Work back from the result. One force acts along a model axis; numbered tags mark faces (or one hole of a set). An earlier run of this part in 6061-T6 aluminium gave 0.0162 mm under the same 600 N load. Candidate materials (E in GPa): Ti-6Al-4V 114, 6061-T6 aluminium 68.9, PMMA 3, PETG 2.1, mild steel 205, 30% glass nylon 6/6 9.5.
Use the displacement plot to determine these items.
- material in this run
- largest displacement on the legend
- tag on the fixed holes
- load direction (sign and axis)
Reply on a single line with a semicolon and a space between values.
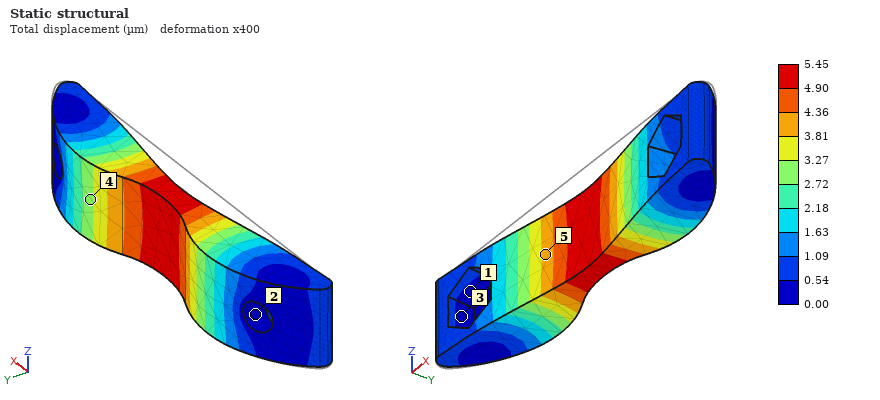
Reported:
mild steel; 5.45 µm; 2; +Y
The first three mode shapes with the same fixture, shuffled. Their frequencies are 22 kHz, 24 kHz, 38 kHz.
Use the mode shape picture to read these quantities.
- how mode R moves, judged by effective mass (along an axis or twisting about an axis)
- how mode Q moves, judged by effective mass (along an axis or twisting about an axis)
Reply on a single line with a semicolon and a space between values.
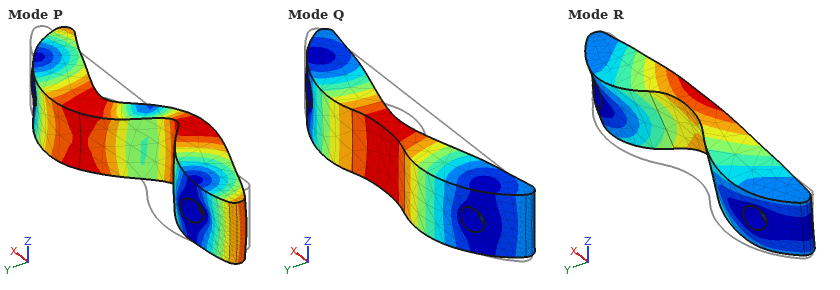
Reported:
along Z; along Y
